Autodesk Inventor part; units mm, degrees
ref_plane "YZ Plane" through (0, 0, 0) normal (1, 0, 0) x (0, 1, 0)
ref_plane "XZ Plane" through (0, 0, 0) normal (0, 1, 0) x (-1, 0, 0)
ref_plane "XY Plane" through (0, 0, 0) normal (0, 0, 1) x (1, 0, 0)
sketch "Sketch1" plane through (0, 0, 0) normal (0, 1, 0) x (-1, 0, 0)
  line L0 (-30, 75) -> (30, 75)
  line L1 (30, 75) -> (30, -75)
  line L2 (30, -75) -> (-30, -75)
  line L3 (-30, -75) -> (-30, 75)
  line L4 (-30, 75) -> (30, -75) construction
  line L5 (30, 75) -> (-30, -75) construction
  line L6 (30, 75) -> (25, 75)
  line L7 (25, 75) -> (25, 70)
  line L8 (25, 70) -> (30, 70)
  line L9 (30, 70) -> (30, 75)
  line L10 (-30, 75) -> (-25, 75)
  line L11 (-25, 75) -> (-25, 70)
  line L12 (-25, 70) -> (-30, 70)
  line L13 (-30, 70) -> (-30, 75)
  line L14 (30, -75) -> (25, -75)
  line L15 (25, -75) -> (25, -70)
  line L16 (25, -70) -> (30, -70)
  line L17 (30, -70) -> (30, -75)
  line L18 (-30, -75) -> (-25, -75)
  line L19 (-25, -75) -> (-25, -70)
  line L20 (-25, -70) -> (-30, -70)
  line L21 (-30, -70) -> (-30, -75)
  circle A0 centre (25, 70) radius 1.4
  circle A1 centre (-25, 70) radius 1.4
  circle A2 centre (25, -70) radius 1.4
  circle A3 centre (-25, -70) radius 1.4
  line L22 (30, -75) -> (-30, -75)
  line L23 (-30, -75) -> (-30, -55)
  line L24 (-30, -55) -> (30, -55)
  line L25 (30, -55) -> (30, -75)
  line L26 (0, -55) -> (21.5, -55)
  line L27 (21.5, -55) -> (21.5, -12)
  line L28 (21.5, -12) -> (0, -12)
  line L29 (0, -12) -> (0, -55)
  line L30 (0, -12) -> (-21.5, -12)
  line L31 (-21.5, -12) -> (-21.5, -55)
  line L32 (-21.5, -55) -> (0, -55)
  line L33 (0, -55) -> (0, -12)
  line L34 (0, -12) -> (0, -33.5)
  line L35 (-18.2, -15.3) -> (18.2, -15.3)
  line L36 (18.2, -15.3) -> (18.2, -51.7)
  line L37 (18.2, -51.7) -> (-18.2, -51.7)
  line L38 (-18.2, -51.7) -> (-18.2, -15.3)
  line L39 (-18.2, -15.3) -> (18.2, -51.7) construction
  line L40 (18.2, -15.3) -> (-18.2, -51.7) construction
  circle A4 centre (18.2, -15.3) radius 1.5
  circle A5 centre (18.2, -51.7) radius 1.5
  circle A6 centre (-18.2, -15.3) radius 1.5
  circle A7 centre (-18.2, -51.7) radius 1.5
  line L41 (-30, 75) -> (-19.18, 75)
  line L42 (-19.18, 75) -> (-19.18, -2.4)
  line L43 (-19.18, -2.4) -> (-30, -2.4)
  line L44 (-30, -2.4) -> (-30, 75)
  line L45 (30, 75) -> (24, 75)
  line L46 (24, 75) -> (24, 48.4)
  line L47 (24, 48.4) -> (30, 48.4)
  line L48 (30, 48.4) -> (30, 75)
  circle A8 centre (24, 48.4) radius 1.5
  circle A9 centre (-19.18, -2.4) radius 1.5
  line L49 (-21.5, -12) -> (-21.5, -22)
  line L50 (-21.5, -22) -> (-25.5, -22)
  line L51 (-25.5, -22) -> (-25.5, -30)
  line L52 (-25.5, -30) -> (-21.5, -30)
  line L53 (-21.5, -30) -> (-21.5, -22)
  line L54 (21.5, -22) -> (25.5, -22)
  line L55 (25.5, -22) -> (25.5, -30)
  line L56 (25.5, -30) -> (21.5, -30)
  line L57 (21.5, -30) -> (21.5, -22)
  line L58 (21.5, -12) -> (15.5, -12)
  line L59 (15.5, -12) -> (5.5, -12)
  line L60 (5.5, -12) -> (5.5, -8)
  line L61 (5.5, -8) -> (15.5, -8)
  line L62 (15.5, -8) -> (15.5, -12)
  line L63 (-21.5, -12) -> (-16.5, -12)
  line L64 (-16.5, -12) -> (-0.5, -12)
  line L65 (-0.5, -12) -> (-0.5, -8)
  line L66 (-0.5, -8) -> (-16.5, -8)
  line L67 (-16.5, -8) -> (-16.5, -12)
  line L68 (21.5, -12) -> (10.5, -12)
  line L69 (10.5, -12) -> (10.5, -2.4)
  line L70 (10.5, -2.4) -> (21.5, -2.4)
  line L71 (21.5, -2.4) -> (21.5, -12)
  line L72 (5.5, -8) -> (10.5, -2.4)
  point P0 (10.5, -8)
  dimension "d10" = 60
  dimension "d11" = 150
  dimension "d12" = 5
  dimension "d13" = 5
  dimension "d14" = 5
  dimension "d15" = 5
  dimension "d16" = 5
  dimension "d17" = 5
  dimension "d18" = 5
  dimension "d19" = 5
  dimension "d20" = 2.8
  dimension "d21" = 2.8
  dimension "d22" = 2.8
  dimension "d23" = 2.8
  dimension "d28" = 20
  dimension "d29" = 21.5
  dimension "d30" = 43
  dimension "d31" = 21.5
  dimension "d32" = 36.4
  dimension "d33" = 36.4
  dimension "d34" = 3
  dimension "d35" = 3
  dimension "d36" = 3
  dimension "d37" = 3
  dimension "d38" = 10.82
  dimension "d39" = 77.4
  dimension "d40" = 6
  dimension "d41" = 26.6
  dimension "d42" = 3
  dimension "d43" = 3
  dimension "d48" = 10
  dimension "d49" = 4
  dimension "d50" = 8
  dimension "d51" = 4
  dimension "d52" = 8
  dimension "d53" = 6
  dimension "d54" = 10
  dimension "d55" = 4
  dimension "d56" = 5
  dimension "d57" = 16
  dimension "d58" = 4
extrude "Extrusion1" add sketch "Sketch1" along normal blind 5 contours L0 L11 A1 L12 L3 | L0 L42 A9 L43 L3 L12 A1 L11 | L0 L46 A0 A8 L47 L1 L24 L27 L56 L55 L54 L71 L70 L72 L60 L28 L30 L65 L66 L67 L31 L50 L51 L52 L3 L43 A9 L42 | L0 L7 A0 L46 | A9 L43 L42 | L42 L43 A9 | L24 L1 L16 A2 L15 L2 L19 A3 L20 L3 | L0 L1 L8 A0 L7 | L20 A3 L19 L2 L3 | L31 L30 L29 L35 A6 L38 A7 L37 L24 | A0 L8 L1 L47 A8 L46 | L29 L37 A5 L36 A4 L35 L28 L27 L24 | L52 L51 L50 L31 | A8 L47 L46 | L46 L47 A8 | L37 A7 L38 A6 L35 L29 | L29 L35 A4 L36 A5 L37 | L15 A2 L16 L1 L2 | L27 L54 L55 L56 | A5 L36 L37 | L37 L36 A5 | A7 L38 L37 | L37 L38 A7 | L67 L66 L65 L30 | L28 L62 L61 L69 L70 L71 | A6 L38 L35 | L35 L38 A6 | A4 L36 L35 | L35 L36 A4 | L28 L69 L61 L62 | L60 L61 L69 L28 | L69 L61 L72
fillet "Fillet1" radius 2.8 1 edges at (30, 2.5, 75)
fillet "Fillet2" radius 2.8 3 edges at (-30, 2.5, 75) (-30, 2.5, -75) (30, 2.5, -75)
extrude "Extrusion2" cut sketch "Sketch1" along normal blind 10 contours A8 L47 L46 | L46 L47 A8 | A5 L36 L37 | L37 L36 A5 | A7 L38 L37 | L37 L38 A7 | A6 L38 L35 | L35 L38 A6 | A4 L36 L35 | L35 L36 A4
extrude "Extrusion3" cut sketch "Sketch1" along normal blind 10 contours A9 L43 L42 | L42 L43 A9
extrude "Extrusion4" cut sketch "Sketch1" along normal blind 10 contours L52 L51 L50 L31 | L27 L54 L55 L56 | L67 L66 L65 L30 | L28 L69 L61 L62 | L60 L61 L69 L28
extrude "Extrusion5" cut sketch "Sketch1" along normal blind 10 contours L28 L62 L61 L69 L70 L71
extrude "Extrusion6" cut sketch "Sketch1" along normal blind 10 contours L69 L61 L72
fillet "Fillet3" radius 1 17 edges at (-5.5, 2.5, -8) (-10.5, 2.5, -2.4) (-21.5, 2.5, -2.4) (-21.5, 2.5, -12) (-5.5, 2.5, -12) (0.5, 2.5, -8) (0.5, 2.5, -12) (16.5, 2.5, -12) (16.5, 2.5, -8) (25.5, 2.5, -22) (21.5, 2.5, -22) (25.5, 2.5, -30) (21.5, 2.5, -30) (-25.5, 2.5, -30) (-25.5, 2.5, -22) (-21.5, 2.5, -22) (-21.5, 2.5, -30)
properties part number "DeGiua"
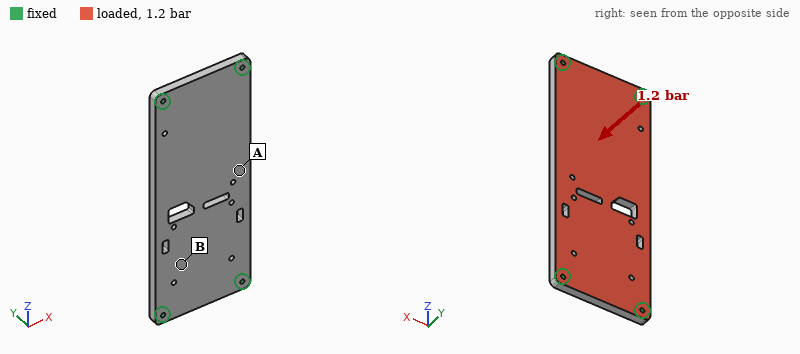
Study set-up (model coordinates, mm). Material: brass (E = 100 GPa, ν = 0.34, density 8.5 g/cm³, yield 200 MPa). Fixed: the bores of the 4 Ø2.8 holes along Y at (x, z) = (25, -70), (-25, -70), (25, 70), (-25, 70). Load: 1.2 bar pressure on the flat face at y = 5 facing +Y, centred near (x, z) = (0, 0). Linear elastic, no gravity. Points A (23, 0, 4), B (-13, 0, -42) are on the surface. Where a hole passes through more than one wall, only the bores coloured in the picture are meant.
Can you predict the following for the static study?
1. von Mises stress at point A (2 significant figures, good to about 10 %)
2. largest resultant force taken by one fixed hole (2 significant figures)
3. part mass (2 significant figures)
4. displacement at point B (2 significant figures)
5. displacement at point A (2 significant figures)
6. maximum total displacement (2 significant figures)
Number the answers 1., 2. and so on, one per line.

1. 29 MPa
2. 260 N
3. 370 g
4. 0.083 mm
5. 0.17 mm
6. 0.18 mm
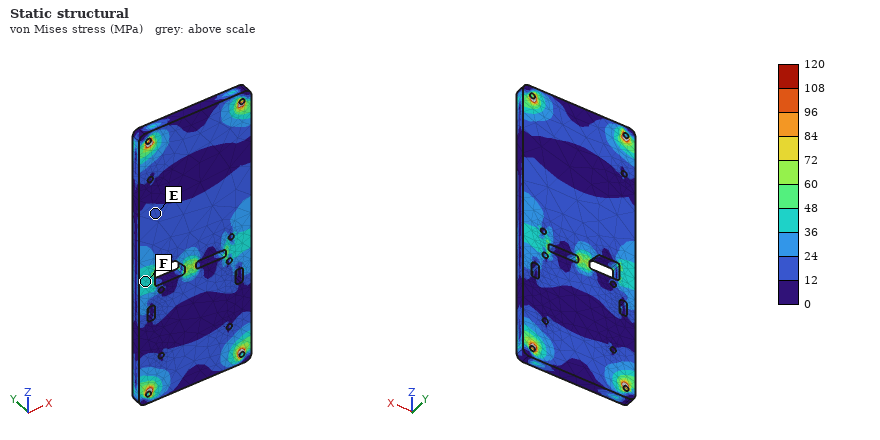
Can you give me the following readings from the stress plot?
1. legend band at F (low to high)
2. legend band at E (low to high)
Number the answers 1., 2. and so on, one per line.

1. 36 to 48 MPa
2. 12 to 24 MPa
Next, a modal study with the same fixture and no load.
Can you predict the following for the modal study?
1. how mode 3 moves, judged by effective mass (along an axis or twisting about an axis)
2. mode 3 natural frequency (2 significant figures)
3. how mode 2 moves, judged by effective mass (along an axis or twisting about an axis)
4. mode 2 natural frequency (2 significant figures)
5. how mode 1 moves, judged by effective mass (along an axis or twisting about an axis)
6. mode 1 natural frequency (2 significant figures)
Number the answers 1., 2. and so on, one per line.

1. twisting about X
2. 2100 Hz
3. twisting about Z
4. 1600 Hz
5. along Y
6. 730 Hz
